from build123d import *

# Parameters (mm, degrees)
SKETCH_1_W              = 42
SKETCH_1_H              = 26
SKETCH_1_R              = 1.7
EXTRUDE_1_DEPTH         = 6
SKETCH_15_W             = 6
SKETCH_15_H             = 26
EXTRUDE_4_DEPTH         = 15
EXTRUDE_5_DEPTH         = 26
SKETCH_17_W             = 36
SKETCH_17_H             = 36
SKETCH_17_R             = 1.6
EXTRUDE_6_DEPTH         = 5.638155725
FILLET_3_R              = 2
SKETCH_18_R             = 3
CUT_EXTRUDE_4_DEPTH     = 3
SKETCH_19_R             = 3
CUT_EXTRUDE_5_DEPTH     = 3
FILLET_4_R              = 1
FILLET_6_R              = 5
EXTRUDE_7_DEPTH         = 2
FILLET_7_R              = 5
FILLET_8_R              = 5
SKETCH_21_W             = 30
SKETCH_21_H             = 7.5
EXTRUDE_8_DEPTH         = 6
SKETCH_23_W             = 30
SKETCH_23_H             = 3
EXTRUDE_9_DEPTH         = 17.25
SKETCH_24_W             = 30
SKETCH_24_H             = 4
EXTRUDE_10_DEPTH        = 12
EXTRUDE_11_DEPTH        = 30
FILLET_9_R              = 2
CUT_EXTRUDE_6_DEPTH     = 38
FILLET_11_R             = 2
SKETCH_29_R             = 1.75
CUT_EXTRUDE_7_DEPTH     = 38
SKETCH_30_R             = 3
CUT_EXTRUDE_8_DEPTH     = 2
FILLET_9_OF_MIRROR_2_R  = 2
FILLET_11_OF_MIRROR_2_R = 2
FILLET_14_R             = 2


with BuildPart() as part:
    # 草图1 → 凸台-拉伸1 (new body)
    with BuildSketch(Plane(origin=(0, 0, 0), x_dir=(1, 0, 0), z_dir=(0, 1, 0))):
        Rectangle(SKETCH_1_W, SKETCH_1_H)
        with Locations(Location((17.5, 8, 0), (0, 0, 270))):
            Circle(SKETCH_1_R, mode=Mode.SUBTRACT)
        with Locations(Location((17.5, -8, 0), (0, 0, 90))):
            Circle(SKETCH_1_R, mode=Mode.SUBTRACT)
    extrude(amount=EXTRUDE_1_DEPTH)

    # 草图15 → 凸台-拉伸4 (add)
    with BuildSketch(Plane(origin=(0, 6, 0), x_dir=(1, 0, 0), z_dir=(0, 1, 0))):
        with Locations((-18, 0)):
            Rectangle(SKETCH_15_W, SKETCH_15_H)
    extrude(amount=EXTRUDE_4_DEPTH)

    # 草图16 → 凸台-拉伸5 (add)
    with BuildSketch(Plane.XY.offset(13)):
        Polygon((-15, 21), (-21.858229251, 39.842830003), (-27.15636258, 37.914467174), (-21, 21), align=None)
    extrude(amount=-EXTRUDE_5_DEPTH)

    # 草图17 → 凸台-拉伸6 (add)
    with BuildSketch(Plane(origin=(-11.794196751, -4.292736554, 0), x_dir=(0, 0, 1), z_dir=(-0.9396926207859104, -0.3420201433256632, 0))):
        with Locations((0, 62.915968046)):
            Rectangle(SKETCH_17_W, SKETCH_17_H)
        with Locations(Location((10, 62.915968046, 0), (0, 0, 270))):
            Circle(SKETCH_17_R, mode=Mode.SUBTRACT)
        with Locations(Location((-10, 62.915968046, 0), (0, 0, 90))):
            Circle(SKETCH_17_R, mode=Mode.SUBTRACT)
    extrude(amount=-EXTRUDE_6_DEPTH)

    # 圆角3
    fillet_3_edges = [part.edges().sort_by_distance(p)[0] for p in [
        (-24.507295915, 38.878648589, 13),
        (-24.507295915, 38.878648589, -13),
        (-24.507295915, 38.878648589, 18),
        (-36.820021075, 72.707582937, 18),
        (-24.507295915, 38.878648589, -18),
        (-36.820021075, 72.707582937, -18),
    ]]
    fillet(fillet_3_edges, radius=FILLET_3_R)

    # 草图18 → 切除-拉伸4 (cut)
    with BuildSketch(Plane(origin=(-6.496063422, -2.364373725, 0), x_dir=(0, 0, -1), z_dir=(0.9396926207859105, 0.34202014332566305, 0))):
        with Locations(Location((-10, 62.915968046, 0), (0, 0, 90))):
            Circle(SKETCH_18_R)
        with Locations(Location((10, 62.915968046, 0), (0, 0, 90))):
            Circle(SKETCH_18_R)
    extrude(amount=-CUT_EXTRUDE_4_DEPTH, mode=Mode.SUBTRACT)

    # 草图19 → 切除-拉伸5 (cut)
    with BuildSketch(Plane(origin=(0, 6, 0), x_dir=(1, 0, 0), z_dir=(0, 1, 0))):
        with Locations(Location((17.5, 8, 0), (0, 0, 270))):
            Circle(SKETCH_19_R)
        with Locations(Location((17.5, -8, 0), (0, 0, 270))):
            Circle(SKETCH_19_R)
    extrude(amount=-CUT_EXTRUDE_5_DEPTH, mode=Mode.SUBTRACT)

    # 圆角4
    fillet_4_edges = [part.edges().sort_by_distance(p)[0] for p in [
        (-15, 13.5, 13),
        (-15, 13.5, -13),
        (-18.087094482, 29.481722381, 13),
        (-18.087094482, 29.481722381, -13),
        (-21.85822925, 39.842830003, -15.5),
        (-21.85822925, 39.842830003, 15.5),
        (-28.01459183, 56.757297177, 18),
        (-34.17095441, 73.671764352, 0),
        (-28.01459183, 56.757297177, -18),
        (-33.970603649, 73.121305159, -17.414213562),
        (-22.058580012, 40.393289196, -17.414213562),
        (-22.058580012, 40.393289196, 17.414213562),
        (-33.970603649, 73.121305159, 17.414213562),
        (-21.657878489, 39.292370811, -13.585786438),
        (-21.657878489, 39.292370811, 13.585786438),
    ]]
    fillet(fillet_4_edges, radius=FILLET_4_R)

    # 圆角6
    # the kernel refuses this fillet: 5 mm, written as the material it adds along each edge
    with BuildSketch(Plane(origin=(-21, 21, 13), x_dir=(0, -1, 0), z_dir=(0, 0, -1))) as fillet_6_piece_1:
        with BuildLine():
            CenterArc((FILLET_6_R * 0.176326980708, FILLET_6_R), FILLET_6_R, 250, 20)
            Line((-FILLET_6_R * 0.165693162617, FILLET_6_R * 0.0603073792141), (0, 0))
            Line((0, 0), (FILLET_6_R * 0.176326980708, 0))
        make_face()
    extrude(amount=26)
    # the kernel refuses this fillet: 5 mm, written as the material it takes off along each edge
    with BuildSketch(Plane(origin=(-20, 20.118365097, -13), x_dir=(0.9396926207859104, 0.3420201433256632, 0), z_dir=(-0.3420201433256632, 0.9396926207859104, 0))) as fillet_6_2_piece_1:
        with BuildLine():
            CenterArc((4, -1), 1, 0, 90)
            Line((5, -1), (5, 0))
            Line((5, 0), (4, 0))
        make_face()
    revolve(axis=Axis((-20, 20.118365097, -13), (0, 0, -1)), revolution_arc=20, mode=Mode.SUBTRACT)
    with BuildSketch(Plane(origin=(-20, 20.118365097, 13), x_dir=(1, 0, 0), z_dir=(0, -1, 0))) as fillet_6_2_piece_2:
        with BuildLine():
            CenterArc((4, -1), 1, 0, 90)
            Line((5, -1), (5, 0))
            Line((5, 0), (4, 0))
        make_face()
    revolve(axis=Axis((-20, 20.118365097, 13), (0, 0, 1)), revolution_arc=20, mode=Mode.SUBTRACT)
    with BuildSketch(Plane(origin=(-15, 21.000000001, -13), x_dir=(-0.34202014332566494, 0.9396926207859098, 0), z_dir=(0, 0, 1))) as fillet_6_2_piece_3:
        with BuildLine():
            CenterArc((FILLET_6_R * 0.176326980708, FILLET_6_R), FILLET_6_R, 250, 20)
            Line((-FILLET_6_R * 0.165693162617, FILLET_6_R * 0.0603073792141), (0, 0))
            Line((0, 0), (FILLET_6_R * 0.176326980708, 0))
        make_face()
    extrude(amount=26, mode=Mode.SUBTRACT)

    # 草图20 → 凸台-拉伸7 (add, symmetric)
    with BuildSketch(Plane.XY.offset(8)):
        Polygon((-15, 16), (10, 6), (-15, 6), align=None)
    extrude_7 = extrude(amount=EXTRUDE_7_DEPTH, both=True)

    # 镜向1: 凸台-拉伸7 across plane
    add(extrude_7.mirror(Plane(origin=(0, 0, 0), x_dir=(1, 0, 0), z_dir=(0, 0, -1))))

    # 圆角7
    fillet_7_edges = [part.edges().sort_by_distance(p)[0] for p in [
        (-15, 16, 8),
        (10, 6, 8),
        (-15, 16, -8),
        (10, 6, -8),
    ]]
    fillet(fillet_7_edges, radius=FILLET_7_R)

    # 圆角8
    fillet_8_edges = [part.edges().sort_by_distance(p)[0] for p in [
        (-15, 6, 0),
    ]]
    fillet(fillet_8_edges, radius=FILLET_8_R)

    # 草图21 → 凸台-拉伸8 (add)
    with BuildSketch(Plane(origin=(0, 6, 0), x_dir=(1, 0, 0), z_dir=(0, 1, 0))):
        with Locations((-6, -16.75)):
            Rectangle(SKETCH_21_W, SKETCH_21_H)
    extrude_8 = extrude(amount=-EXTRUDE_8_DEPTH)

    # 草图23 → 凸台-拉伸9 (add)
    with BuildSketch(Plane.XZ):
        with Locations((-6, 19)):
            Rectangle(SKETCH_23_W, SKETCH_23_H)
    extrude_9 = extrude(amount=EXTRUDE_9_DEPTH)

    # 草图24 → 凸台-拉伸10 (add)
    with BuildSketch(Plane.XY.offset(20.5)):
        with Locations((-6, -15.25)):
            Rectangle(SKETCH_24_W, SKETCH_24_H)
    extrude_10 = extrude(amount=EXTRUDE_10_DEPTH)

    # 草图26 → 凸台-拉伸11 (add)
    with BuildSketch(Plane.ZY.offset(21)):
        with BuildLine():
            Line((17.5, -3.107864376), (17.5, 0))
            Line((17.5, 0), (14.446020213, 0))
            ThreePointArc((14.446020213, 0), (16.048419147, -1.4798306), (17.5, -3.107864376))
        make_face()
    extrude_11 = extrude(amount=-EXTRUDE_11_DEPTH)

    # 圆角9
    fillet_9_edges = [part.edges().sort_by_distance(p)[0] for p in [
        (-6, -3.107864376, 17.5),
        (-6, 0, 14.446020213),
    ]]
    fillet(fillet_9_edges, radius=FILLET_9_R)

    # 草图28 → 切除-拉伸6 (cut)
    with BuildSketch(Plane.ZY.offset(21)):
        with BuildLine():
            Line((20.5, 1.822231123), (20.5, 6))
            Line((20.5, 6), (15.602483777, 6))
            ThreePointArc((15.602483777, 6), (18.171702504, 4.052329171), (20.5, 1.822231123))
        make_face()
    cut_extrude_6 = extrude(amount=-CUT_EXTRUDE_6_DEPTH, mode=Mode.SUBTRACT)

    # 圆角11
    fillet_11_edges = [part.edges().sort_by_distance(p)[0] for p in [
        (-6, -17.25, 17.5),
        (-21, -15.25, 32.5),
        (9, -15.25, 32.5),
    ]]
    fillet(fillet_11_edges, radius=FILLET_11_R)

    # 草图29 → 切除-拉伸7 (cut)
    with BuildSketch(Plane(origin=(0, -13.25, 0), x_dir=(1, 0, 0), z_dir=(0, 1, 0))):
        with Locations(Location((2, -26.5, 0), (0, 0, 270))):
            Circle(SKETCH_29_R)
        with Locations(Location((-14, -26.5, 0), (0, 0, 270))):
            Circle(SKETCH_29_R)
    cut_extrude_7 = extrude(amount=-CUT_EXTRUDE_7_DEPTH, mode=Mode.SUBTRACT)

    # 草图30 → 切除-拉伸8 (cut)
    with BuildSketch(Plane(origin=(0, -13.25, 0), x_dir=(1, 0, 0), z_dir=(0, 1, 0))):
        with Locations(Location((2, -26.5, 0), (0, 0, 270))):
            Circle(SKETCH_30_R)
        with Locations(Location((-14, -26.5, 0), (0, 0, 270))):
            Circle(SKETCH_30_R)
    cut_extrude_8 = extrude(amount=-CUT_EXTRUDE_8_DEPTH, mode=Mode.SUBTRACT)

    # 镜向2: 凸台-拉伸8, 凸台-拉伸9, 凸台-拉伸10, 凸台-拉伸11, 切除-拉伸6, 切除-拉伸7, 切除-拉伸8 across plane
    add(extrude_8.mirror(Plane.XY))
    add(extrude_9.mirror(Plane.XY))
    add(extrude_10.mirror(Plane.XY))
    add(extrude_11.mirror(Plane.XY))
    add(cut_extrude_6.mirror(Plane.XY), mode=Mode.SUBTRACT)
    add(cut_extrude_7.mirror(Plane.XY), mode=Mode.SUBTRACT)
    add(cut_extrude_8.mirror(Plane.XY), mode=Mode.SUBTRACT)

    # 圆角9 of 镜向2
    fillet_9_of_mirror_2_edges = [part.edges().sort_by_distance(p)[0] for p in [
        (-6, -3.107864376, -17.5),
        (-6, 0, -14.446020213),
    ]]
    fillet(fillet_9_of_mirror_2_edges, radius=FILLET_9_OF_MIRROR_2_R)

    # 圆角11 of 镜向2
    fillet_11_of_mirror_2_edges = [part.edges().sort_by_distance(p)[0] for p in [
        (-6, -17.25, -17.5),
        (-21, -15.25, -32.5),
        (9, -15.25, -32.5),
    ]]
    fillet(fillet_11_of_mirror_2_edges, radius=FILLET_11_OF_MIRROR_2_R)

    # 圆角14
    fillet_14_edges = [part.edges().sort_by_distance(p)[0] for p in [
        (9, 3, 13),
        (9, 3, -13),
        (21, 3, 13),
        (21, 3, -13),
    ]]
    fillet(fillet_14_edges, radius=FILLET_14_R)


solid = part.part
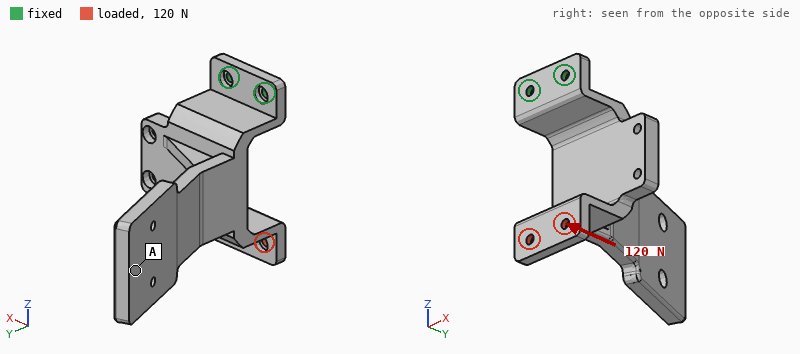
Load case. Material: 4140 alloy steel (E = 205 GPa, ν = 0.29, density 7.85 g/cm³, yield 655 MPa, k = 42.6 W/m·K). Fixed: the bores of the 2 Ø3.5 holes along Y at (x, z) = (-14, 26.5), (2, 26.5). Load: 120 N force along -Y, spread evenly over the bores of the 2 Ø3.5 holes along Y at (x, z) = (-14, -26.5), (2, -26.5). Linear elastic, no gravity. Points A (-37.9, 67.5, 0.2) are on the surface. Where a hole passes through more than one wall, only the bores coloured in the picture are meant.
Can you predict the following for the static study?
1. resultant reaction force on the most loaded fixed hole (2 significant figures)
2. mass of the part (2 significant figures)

60 N
220 g
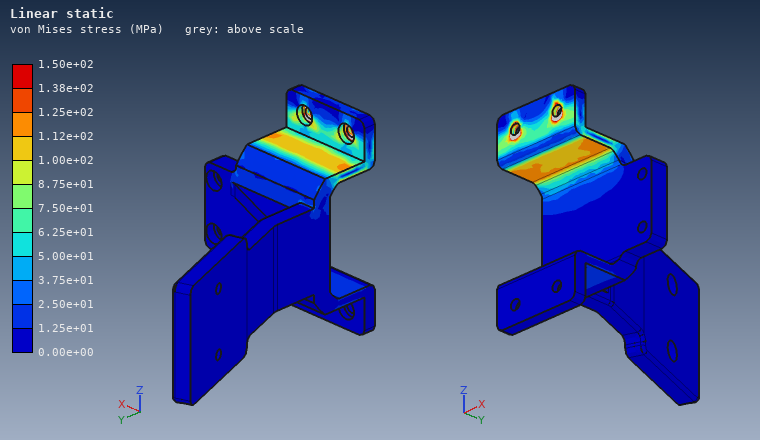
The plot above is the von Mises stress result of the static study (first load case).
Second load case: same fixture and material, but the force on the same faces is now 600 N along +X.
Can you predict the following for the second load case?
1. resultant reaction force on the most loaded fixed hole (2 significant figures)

1.7 kN
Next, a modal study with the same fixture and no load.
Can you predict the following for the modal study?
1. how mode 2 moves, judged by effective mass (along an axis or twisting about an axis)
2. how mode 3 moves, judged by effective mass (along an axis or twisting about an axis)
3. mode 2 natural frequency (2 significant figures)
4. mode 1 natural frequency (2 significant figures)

along X
along X
670 Hz
200 Hz
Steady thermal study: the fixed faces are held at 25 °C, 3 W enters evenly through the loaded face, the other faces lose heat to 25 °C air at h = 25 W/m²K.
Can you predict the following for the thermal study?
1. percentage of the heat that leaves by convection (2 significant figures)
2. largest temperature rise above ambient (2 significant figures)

74 %
25 K
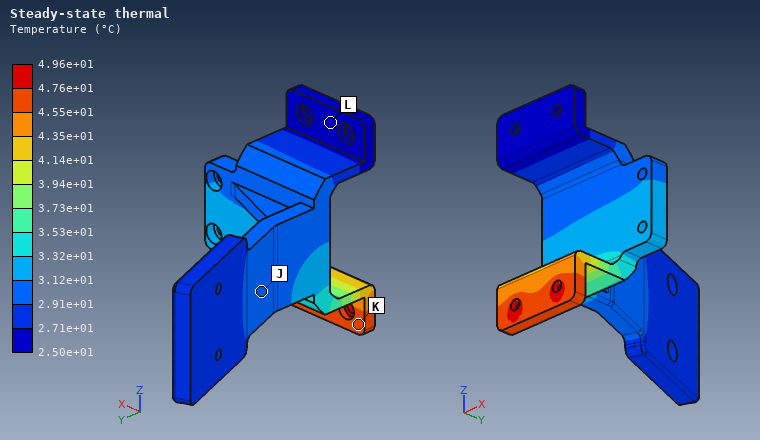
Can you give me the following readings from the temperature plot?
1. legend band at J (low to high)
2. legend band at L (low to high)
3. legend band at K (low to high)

2.91e+01 to 3.12e+01 °C
2.50e+01 to 2.71e+01 °C
4.55e+01 to 4.76e+01 °C
